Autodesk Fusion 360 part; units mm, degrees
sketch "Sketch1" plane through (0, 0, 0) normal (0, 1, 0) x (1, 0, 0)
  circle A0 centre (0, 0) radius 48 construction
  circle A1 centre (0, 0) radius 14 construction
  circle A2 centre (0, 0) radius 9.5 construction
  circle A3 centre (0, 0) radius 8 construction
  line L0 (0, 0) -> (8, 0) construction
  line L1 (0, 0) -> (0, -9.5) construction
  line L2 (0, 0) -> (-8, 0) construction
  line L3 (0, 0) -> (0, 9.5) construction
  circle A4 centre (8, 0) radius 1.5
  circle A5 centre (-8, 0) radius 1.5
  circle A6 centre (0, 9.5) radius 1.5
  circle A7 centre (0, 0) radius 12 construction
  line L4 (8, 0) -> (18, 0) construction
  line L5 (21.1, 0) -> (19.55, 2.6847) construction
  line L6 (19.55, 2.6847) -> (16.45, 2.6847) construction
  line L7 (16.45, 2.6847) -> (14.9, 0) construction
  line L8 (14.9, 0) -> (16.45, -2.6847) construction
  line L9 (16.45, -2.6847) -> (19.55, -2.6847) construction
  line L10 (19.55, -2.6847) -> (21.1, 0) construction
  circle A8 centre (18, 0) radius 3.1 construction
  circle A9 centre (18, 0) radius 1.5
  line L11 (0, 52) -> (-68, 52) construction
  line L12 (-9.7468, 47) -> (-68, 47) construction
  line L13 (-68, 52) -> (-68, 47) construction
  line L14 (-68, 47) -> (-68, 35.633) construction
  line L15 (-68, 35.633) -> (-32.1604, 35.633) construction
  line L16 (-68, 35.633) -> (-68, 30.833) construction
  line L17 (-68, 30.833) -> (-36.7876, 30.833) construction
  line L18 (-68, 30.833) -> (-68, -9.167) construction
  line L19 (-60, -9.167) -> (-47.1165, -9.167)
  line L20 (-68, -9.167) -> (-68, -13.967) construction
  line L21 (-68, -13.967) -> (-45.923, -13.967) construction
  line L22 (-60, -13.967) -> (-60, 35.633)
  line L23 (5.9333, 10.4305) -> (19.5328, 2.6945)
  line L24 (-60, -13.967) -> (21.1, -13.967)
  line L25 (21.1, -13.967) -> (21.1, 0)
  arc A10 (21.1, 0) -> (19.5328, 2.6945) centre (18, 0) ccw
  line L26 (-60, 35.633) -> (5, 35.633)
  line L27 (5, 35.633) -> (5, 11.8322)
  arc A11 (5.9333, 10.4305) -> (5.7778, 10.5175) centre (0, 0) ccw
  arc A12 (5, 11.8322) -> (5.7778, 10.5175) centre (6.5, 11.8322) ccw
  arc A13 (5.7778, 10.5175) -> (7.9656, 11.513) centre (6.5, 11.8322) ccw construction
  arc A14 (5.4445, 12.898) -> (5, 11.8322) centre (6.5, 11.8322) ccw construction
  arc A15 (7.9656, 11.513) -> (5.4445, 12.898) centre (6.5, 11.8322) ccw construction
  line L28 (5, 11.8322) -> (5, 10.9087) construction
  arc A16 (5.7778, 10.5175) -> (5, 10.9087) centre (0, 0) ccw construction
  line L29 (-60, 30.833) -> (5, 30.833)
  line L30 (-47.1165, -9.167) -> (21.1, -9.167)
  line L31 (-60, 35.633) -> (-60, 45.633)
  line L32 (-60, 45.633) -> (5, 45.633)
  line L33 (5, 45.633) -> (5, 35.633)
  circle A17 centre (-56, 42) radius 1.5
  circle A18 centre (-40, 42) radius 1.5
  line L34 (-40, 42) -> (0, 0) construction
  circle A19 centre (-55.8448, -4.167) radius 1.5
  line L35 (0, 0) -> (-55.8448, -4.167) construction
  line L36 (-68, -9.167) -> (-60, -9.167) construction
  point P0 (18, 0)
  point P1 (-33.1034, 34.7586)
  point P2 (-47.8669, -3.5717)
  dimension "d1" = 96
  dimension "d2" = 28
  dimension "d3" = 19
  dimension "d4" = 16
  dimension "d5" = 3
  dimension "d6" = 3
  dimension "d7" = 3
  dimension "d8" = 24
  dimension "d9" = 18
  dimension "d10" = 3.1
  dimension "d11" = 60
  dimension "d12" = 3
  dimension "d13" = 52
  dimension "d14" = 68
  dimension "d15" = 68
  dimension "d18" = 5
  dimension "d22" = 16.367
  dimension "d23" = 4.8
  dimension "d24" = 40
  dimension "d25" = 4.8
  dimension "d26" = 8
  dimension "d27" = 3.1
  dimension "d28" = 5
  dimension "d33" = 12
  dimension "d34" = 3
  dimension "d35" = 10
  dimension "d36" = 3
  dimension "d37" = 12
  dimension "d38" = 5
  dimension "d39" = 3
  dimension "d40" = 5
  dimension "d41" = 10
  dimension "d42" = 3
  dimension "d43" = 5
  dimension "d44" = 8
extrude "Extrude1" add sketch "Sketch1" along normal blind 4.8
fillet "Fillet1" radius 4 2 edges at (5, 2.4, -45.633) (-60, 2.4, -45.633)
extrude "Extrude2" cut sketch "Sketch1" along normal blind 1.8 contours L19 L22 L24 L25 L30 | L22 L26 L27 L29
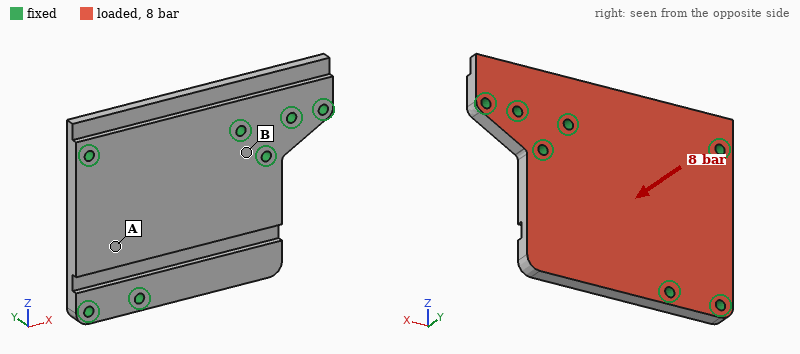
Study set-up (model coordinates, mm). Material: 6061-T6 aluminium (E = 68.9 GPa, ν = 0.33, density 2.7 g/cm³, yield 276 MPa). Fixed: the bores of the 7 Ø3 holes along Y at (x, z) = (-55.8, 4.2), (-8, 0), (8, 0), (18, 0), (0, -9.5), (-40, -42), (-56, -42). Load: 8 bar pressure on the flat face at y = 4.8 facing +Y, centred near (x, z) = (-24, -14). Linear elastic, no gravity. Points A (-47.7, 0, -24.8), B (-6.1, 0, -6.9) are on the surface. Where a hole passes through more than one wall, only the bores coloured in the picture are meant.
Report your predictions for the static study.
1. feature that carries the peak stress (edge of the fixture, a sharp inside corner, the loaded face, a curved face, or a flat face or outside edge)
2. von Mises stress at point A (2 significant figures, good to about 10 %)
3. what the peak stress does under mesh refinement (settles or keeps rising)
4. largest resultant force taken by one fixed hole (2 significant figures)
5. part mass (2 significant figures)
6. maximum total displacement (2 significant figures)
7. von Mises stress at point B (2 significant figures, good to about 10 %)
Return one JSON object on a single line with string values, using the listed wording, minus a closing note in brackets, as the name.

{"feature that carries the peak stress": "edge of the fixture", "von Mises stress at point A": "17 MPa", "what the peak stress does under mesh refinement": "keeps rising", "largest resultant force taken by one fixed hole": "860 N", "part mass": "50 g", "maximum total displacement": "0.15 mm", "von Mises stress at point B": "38 MPa"}
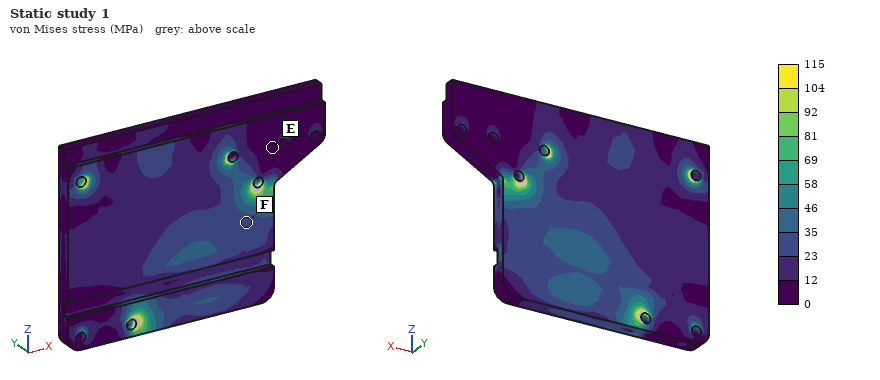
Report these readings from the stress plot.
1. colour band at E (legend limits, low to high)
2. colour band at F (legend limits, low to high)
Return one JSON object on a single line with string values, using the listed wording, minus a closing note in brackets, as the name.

{"colour band at E": "0 to 12 MPa", "colour band at F": "23 to 35 MPa"}
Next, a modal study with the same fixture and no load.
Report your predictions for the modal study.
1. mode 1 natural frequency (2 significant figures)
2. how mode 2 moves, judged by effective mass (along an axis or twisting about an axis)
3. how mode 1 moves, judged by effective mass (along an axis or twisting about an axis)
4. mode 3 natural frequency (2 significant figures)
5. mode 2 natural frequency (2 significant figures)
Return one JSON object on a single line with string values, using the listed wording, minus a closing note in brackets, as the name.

{"mode 1 natural frequency": "4600 Hz", "how mode 2 moves, judged by effective mass": "along Y", "how mode 1 moves, judged by effective mass": "along Y", "mode 3 natural frequency": "10 kHz", "mode 2 natural frequency": "8200 Hz"}
